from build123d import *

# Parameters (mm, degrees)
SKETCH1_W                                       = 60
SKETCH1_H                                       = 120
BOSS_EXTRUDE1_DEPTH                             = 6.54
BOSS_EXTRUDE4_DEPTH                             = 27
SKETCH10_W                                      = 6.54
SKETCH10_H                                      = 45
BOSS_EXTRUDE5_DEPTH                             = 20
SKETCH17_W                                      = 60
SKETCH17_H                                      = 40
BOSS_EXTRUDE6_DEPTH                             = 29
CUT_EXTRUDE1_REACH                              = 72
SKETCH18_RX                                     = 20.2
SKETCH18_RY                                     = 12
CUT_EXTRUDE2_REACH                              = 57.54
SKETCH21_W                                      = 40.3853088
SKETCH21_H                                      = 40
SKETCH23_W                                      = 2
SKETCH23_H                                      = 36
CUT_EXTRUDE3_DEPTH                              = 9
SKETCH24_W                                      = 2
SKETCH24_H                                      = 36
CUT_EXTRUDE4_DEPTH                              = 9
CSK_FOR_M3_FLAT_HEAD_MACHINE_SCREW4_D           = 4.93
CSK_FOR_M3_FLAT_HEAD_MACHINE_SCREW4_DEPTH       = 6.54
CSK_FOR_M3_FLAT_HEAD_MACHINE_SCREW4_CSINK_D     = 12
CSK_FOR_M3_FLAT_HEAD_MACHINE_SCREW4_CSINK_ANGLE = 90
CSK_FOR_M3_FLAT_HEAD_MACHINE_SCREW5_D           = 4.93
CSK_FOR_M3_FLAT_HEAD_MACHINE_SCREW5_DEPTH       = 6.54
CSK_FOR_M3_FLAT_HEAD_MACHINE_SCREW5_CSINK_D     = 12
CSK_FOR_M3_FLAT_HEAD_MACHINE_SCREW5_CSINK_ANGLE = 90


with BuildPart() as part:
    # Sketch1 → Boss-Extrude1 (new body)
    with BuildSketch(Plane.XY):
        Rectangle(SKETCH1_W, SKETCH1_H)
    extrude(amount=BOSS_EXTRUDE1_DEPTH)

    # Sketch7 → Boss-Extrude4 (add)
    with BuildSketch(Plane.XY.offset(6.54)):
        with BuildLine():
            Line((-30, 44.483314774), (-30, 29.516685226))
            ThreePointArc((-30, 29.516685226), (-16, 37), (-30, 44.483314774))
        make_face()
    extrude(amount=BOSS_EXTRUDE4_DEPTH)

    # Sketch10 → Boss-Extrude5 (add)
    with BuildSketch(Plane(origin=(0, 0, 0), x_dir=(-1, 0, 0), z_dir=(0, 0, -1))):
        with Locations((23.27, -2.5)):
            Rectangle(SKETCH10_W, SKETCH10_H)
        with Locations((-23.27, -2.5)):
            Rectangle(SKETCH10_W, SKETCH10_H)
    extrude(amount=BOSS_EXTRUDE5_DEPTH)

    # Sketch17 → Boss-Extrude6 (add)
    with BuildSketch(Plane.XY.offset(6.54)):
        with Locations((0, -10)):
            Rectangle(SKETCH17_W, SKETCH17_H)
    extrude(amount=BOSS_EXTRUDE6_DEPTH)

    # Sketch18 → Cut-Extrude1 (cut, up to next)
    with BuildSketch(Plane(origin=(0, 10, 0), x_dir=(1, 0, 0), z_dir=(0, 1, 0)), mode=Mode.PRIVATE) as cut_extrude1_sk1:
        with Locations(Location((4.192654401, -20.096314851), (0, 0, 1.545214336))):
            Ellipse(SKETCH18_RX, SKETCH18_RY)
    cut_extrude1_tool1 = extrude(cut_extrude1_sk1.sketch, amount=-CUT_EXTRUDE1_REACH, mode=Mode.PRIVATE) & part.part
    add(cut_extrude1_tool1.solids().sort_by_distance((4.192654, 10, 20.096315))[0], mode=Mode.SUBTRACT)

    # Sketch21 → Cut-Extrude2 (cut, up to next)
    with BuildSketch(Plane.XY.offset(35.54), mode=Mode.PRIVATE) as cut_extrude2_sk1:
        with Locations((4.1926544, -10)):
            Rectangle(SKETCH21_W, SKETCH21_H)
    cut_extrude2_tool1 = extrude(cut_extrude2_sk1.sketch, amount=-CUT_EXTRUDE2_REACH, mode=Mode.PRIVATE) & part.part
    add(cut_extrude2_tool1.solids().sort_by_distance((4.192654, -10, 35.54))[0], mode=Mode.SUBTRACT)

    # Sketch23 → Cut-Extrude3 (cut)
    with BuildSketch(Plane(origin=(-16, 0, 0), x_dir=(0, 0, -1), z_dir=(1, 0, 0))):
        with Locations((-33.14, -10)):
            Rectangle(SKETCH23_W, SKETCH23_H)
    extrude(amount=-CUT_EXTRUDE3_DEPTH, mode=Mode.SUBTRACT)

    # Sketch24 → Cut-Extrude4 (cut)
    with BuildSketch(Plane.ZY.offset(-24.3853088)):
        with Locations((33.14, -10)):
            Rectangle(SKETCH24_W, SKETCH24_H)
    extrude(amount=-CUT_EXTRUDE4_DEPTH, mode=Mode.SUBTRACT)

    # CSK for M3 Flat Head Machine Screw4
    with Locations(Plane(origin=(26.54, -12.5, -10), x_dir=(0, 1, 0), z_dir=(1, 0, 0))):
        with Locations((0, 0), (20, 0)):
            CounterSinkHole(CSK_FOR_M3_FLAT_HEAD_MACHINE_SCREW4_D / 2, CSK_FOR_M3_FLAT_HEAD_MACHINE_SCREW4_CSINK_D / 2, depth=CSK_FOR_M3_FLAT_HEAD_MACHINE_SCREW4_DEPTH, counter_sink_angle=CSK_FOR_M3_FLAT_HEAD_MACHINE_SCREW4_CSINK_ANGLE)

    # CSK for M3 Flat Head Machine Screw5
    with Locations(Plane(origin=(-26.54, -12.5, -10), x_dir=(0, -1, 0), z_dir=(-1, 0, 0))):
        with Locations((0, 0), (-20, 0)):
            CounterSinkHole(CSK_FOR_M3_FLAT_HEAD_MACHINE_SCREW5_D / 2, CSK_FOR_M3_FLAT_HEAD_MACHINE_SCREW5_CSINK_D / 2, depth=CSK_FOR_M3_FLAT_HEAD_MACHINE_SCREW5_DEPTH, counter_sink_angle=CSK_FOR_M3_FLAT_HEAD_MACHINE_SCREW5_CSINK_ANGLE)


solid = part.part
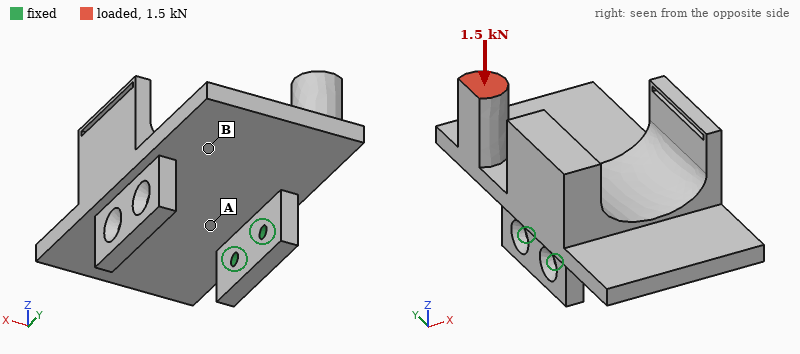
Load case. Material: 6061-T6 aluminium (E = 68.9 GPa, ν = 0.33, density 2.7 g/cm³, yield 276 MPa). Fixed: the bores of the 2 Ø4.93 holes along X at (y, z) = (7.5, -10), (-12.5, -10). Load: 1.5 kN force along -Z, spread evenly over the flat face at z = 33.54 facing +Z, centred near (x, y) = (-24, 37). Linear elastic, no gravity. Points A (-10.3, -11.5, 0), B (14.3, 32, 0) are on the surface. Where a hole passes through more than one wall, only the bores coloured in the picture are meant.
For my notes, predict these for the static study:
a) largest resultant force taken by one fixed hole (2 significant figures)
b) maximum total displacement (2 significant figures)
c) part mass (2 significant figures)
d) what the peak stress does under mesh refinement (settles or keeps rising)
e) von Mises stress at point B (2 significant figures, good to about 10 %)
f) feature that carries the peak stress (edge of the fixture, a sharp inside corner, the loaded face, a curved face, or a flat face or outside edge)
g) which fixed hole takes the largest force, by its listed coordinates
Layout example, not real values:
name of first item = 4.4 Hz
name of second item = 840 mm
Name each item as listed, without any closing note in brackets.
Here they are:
largest resultant force taken by one fixed hole = 3.4 kN
maximum total displacement = 0.31 mm
part mass = 250 g
what the peak stress does under mesh refinement = keeps rising
von Mises stress at point B = 26 MPa
feature that carries the peak stress = edge of the fixture
which fixed hole takes the largest force, by its listed coordinates = (7.5, -10)
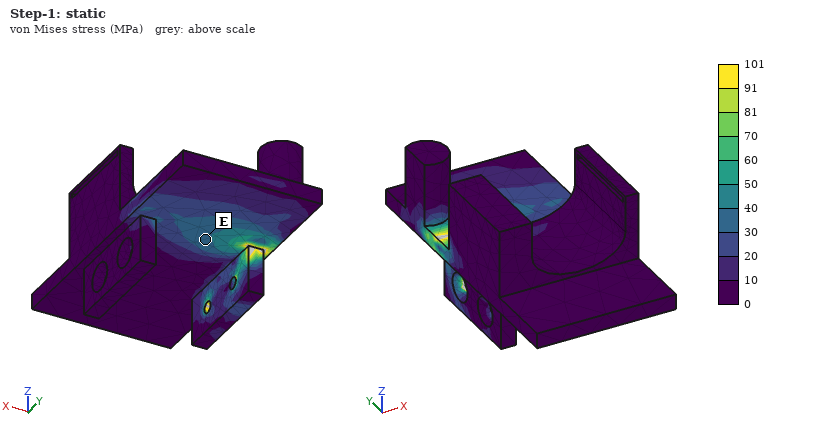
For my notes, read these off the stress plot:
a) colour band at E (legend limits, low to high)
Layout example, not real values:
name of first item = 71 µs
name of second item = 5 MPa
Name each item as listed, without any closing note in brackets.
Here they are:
colour band at E = 30 to 40 MPa
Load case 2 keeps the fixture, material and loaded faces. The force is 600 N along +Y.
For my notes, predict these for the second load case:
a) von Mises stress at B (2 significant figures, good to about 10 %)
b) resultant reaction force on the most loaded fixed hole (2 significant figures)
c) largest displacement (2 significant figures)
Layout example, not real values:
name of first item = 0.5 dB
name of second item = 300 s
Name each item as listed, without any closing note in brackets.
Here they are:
von Mises stress at B = 23 MPa
resultant reaction force on the most loaded fixed hole = 1.2 kN
largest displacement = 0.26 mm
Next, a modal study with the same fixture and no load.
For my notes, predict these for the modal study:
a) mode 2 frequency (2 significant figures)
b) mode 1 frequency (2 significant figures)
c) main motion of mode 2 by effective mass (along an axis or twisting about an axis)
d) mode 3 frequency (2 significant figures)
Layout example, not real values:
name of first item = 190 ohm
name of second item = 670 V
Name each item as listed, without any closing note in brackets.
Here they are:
mode 2 frequency = 1100 Hz
mode 1 frequency = 560 Hz
main motion of mode 2 by effective mass = along Y
mode 3 frequency = 1600 Hz
